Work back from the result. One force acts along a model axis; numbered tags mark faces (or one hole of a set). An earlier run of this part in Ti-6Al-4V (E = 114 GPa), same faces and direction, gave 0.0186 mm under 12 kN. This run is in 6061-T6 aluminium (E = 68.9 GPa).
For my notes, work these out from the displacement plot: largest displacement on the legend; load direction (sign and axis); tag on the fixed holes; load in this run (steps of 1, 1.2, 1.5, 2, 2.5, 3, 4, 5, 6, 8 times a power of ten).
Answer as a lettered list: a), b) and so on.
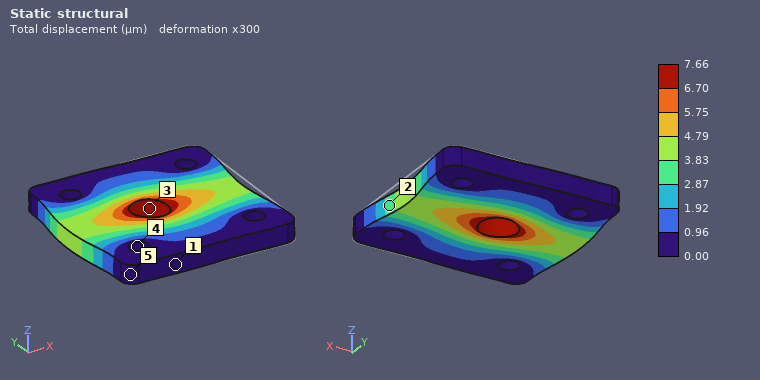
a) 7.66 µm
b) -X
c) 4
d) 3 kN
